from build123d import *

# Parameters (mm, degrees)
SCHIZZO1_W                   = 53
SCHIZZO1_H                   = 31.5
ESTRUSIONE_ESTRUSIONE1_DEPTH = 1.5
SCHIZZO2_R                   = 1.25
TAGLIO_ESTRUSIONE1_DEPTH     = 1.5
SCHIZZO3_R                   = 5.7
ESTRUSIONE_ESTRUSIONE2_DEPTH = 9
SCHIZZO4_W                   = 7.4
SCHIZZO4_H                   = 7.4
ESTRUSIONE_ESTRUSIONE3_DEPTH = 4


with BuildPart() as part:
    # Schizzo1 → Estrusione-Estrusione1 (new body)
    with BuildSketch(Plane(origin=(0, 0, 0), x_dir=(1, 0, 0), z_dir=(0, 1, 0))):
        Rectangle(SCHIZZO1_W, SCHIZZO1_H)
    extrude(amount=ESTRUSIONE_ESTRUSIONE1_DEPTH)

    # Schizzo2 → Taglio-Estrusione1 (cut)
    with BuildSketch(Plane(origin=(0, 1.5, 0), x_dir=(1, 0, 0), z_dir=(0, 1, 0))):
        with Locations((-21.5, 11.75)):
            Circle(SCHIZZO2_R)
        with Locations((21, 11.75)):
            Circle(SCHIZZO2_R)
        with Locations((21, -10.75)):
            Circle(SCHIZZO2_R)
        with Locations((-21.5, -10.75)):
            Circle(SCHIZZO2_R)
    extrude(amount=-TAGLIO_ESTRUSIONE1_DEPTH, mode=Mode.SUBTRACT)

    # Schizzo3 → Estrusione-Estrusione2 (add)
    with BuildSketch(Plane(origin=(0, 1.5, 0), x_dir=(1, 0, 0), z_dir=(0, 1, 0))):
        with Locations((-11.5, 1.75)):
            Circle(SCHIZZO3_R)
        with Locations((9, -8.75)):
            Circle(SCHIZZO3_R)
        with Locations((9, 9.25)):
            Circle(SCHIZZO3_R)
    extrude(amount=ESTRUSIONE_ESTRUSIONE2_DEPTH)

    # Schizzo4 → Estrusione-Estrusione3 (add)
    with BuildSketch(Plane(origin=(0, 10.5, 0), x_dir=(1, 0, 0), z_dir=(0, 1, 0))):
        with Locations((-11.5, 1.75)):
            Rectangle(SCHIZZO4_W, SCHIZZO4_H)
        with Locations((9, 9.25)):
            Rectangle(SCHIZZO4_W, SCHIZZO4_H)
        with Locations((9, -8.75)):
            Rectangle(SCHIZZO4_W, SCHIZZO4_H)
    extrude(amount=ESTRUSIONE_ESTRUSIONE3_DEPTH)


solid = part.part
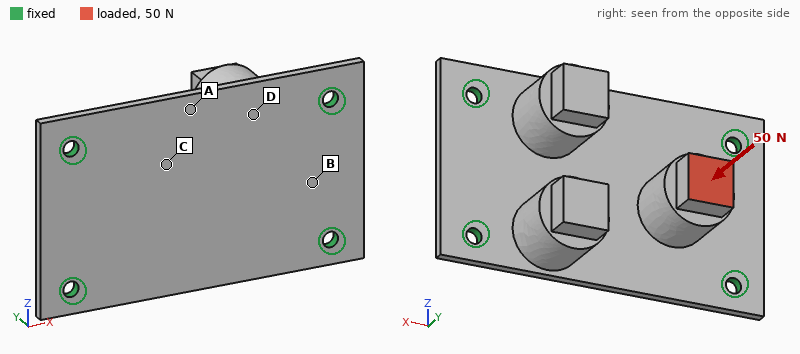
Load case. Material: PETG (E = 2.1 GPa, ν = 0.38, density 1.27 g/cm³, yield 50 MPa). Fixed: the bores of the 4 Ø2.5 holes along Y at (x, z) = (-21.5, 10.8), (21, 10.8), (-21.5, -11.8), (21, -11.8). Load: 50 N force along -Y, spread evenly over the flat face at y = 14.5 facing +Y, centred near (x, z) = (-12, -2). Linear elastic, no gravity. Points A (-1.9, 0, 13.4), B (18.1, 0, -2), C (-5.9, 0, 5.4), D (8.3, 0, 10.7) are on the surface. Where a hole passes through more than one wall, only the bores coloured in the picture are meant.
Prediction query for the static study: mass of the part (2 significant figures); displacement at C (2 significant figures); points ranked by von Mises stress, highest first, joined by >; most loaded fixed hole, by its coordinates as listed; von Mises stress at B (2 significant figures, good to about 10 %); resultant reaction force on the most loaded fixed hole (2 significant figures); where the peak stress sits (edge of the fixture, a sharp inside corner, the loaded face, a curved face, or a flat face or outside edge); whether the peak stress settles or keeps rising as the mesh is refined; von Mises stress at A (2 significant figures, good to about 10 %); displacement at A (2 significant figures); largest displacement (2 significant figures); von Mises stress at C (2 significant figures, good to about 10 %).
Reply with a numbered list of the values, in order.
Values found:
1. 7.5 g
2. 0.54 mm
3. C > A > B > D
4. (-21.5, -11.8)
5. 3.5 MPa
6. 23 N
7. edge of the fixture
8. keeps rising
9. 7.1 MPa
10. 0.44 mm
11. 0.68 mm
12. 9.4 MPa
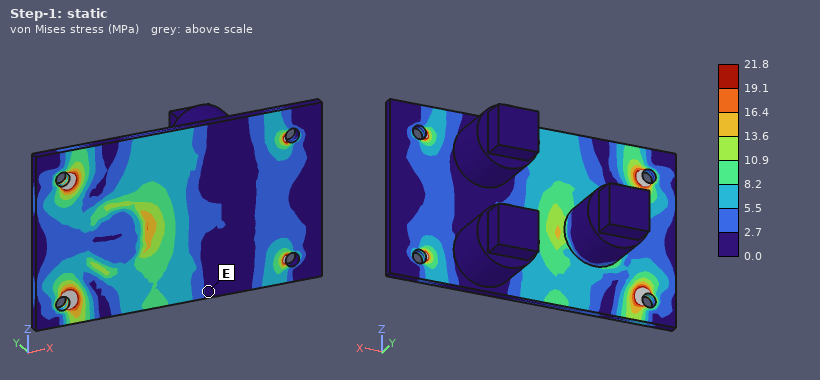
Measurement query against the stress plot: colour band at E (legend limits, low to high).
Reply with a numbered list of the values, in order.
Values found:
1. 0.0 to 2.7 MPa
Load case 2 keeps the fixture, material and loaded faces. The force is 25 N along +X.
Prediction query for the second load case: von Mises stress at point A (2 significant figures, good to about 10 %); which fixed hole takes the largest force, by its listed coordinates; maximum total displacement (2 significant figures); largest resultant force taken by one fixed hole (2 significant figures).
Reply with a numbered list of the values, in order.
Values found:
1. 5.9 MPa
2. (-21.5, -11.8)
3. 0.67 mm
4. 10 N
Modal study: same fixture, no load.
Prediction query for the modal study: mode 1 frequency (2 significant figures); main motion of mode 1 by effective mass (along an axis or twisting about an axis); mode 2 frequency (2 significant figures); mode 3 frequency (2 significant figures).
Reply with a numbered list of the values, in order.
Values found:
1. 620 Hz
2. along Y
3. 1000 Hz
4. 1200 Hz
